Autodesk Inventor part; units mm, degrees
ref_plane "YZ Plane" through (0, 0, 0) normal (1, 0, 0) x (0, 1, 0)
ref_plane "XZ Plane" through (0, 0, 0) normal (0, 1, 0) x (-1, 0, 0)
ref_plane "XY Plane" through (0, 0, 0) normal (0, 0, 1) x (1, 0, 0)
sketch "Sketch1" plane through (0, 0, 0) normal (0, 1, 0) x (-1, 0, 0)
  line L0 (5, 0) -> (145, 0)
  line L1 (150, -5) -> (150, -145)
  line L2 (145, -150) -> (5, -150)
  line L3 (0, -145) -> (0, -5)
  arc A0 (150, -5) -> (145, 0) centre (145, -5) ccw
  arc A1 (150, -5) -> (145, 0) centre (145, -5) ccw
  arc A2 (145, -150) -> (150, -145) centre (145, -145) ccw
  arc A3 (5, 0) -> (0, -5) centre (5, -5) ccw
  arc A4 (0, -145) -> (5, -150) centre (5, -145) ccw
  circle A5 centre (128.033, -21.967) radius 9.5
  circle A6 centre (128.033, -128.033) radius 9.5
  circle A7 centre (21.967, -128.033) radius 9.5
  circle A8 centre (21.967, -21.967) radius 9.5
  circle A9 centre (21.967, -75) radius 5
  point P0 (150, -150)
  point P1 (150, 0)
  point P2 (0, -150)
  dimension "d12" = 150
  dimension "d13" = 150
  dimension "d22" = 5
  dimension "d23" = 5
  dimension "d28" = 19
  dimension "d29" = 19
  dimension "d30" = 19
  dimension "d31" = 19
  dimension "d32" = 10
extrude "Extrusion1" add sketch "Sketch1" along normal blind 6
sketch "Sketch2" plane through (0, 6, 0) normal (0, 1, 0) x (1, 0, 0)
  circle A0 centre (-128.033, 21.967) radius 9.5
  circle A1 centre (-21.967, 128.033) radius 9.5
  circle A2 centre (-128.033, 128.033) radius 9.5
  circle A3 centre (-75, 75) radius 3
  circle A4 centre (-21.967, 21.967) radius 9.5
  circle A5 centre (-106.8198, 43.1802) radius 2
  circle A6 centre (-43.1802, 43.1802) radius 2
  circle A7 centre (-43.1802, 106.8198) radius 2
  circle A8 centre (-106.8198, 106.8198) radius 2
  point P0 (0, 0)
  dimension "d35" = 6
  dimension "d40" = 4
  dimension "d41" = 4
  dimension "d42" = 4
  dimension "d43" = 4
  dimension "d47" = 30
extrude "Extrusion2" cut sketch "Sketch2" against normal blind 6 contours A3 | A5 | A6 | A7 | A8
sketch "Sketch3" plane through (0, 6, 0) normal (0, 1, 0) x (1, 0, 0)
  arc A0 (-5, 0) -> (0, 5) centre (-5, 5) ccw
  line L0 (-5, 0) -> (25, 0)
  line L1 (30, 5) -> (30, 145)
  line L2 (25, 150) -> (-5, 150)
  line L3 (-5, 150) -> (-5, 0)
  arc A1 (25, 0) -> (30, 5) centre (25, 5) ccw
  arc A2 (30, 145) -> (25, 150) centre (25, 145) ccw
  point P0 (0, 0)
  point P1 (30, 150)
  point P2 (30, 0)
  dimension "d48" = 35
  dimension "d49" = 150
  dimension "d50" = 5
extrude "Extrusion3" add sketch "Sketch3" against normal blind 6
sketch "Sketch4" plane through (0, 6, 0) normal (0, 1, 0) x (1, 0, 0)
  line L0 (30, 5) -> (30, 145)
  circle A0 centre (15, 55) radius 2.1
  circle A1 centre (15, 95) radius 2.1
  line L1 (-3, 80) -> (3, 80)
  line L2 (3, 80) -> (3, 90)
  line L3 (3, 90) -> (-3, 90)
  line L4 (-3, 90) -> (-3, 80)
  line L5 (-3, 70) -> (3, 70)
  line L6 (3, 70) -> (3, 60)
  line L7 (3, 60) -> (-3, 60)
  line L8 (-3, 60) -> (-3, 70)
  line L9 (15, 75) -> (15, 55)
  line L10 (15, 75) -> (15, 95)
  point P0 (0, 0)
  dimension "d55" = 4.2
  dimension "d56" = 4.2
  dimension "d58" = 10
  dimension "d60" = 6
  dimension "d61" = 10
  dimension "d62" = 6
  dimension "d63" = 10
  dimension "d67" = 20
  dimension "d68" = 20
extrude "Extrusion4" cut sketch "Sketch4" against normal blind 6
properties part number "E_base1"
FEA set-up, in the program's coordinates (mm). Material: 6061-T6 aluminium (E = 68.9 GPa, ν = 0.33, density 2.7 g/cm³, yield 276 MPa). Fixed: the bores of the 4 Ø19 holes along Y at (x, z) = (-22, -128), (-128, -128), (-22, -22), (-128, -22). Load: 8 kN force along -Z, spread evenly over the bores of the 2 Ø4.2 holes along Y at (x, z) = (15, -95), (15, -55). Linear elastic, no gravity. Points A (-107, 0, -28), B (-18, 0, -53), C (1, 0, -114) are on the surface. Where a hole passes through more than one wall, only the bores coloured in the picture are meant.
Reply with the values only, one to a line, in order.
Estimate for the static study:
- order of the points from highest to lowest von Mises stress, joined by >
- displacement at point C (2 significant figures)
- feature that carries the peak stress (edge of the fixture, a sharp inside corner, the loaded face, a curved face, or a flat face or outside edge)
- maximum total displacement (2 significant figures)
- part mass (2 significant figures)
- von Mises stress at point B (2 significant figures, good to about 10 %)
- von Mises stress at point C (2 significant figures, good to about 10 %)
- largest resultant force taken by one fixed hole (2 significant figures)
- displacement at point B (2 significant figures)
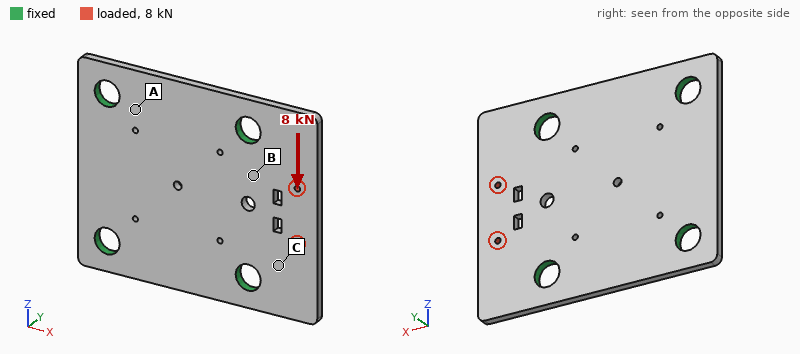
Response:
C > B > A
9.7 µm
the loaded face
23 µm
410 g
12 MPa
22 MPa
4.5 kN
4.1 µm
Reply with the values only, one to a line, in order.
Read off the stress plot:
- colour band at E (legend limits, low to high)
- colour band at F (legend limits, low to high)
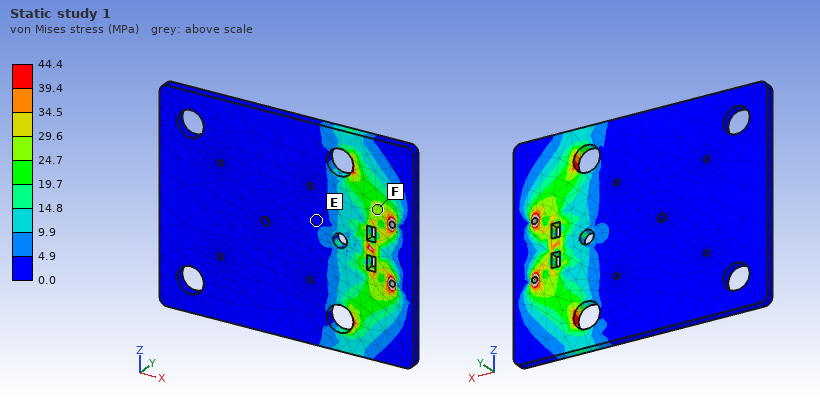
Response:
0.0 to 4.9 MPa
24.7 to 29.6 MPa
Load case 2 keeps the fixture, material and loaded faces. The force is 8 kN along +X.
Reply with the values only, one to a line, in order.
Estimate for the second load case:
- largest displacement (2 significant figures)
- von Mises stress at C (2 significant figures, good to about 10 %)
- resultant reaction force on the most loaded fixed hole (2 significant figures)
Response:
20 µm
16 MPa
3.5 kN
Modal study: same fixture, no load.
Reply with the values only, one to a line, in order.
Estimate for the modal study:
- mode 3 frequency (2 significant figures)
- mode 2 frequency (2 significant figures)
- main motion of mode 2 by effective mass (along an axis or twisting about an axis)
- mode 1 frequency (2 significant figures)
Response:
2900 Hz
2500 Hz
along Y
1900 Hz
